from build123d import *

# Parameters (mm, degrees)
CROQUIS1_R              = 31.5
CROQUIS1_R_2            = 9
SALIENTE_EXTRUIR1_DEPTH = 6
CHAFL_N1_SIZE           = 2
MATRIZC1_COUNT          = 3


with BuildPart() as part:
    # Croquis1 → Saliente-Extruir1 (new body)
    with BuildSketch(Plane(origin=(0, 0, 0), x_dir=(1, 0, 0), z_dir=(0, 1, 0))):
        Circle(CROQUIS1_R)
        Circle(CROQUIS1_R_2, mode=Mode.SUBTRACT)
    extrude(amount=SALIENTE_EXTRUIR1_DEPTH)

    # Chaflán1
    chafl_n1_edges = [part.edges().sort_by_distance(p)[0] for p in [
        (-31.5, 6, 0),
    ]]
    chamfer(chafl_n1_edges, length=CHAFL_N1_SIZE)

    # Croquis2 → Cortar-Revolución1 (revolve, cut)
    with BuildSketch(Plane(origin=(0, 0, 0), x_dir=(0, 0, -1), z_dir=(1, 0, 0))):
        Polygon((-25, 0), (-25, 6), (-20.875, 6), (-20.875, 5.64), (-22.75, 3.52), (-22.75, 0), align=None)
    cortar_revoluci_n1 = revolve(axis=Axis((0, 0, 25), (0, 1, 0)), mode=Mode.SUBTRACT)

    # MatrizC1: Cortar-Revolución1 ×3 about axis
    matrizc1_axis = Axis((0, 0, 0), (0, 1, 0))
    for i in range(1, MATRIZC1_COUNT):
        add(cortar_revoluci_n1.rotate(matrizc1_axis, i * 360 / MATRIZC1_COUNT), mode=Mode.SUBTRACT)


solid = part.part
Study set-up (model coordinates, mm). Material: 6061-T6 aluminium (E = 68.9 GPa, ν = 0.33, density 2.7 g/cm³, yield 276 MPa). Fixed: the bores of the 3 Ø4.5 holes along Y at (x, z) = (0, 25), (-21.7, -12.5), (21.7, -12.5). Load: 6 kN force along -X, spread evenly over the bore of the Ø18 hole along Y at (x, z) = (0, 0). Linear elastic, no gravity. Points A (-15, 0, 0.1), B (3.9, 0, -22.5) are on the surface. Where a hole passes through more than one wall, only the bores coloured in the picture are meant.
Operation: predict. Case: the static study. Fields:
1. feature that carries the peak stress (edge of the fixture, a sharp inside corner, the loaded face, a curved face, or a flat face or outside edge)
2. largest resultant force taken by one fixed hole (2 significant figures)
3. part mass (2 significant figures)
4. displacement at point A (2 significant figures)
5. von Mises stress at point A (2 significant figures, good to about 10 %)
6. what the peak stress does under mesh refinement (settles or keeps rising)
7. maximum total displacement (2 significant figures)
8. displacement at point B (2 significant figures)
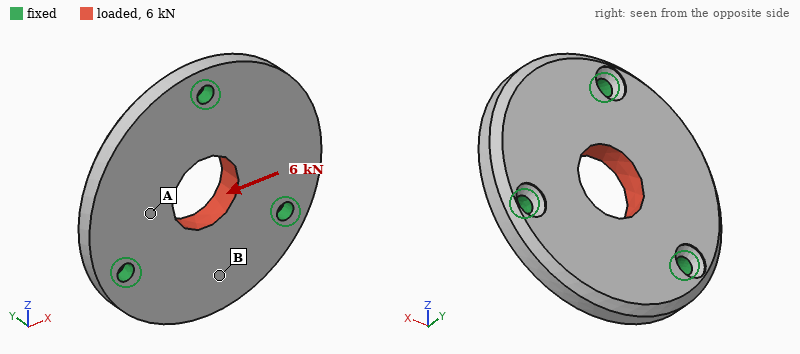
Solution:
edge of the fixture
2.0 kN
44 g
7.0 µm
18 MPa
keeps rising
11 µm
3.2 µm
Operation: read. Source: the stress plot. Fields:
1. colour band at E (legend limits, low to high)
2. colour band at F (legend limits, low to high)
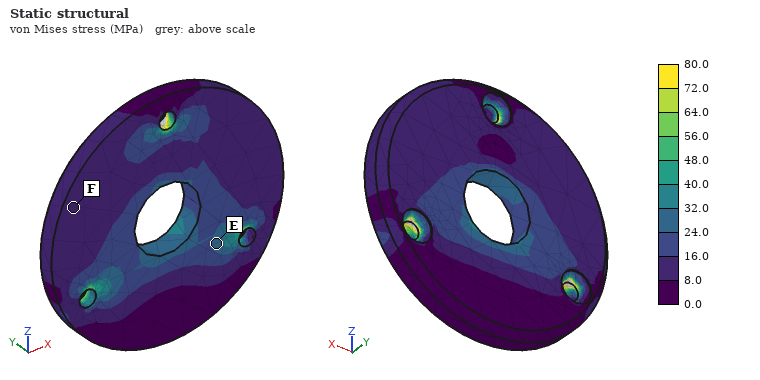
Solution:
24.0 to 32.0 MPa
8.0 to 16.0 MPa
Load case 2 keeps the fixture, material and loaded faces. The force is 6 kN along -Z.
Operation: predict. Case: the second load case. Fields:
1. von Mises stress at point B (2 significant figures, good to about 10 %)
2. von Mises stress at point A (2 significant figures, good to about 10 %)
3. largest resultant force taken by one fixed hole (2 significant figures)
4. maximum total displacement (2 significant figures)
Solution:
13 MPa
16 MPa
2.0 kN
12 µm
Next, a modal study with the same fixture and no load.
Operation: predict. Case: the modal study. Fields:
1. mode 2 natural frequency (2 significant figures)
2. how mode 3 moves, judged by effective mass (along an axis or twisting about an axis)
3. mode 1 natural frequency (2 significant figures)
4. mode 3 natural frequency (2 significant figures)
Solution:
8200 Hz
along Y
8200 Hz
10 kHz
